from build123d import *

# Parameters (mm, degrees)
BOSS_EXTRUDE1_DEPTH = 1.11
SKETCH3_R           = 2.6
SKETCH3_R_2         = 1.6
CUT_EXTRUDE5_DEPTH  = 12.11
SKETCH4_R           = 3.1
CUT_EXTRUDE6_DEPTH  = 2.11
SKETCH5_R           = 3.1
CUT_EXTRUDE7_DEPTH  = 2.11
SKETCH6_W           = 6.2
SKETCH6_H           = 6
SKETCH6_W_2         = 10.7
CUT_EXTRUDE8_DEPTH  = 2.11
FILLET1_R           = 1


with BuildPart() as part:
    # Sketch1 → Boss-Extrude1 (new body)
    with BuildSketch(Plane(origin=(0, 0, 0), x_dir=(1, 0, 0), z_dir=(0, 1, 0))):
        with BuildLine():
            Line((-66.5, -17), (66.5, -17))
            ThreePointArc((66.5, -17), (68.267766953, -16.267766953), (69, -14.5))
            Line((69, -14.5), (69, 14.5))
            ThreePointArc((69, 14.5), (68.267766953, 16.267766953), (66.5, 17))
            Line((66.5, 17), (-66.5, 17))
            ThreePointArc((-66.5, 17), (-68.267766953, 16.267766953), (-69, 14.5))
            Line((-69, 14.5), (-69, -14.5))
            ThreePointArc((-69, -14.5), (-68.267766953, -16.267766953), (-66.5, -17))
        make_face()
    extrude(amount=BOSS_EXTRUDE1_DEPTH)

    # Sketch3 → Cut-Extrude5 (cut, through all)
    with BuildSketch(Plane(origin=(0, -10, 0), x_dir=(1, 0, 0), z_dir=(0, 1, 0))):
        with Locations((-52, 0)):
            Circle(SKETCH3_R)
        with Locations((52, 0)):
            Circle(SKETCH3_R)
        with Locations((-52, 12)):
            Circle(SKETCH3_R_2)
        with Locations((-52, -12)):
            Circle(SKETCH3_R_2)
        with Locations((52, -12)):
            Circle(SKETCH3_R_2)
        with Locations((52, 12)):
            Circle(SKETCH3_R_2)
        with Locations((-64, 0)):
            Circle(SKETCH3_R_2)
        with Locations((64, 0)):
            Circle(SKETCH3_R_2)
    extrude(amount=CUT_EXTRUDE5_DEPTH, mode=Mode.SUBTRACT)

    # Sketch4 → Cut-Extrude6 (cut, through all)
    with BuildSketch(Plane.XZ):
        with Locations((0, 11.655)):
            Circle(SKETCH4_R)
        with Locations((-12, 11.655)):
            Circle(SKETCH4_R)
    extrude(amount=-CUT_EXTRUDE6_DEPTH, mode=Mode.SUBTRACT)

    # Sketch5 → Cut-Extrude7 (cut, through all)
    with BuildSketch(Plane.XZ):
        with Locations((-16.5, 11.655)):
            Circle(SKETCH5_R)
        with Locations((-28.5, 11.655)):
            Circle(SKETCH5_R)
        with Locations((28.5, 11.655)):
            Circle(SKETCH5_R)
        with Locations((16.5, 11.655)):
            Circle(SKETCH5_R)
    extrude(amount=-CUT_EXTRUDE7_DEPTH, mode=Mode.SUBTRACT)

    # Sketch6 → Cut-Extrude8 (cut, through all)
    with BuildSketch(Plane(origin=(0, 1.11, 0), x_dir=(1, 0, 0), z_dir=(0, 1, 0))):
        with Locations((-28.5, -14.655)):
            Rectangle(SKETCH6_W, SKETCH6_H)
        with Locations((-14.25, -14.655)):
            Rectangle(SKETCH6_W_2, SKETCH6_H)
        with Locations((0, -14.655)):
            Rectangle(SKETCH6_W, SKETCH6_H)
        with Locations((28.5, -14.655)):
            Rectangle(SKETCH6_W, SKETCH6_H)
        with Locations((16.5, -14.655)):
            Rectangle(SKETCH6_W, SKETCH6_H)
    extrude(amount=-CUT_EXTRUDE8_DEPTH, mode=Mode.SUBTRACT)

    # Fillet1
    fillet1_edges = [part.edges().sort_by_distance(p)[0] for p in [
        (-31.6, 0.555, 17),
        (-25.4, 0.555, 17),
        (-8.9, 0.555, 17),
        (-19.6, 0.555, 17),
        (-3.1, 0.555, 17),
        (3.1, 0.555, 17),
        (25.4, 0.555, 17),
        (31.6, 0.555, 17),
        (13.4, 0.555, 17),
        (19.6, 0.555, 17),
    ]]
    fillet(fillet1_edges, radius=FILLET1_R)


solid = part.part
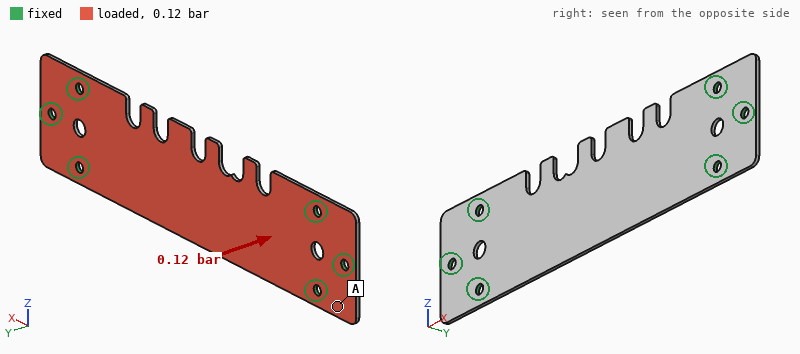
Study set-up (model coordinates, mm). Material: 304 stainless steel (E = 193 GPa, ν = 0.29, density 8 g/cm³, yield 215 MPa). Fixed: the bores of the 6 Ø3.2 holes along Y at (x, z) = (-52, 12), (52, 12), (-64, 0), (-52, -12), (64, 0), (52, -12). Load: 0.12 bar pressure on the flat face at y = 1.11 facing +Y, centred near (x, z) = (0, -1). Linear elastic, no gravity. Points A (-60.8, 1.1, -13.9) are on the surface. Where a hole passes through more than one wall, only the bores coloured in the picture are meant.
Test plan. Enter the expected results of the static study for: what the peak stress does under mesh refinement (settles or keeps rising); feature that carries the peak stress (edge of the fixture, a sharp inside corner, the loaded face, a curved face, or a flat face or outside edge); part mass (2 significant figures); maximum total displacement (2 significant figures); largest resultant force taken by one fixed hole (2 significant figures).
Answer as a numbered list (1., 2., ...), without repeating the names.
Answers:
1. keeps rising
2. edge of the fixture
3. 38 g
4. 0.18 mm
5. 15 N
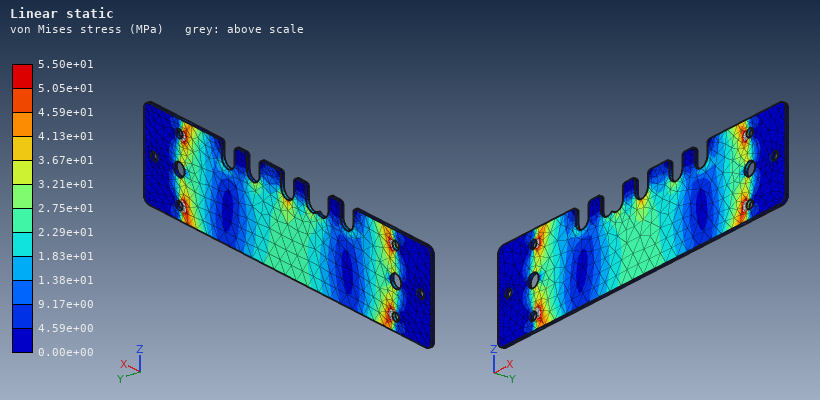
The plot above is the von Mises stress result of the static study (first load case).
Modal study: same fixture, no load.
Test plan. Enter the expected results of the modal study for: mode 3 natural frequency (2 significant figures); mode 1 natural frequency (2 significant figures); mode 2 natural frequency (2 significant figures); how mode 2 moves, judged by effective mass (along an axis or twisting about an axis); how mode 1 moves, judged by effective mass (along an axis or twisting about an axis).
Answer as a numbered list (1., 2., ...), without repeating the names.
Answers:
1. 1400 Hz
2. 520 Hz
3. 1200 Hz
4. twisting about X
5. along Y
